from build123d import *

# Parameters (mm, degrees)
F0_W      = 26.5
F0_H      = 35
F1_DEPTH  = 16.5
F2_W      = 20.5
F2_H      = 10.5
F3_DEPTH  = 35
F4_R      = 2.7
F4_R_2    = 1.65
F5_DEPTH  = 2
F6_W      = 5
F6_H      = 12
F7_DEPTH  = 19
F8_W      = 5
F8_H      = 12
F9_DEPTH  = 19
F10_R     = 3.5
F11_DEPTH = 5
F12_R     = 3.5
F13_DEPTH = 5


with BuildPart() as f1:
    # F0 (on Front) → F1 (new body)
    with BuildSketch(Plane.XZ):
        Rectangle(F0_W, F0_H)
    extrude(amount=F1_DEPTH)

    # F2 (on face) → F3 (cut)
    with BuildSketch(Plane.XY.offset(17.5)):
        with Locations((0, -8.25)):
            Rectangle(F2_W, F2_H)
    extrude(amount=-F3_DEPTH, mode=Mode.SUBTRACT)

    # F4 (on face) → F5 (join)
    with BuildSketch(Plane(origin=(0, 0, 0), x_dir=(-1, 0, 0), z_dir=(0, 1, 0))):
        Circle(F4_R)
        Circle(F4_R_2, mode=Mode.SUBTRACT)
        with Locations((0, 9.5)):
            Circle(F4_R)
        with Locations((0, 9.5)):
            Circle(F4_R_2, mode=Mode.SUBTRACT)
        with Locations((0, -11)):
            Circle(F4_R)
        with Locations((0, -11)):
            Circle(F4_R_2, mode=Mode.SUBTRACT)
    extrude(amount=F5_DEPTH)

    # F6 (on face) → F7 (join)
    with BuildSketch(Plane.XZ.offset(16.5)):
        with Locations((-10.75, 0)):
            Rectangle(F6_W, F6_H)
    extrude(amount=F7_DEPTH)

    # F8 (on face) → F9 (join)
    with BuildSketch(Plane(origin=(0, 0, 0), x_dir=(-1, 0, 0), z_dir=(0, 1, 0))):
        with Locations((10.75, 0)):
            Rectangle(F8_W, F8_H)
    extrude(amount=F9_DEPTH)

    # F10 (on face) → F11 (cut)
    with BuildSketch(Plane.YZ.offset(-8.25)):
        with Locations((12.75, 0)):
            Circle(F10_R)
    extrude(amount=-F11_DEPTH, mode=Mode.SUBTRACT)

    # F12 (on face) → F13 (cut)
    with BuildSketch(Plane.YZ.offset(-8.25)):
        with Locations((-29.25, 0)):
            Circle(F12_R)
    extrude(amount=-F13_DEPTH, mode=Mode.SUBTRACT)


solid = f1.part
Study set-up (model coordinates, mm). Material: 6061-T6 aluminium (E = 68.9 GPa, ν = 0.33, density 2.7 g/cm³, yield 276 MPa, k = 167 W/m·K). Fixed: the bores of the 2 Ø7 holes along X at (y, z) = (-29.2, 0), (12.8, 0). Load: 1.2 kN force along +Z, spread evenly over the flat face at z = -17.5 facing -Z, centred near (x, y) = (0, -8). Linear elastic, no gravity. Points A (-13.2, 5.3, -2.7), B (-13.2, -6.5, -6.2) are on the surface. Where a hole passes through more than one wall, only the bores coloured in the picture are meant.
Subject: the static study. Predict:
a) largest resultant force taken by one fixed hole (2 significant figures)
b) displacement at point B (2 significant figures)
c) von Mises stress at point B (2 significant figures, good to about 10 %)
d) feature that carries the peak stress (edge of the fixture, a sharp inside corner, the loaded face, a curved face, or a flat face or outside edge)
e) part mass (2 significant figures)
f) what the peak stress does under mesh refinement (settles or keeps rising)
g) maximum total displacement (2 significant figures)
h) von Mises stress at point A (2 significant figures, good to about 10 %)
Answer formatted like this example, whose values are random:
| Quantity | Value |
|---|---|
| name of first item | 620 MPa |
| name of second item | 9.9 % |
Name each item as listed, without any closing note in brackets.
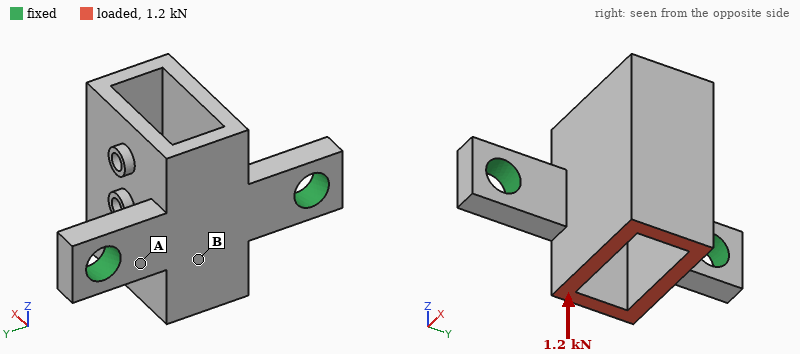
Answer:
| Quantity | Value |
|---|---|
| largest resultant force taken by one fixed hole | 600 N |
| displacement at point B | 0.041 mm |
| von Mises stress at point B | 21 MPa |
| feature that carries the peak stress | edge of the fixture |
| part mass | 26 g |
| what the peak stress does under mesh refinement | keeps rising |
| maximum total displacement | 0.21 mm |
| von Mises stress at point A | 86 MPa |
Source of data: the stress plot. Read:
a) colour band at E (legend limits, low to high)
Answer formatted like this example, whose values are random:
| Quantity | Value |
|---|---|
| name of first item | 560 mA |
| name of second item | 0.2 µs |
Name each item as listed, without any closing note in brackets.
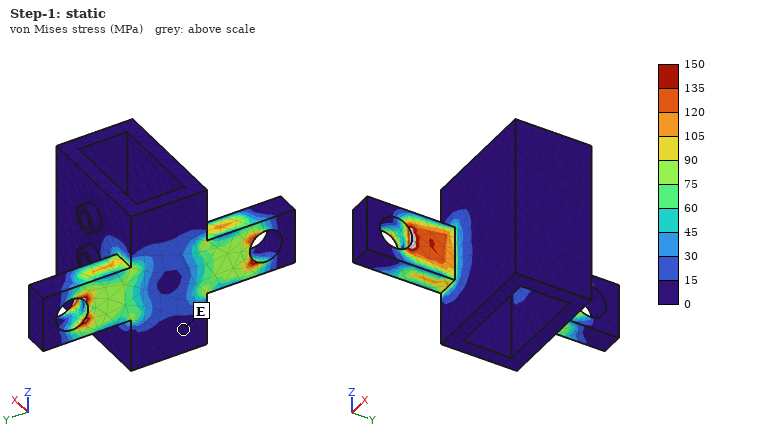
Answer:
| Quantity | Value |
|---|---|
| colour band at E | 0 to 15 MPa |
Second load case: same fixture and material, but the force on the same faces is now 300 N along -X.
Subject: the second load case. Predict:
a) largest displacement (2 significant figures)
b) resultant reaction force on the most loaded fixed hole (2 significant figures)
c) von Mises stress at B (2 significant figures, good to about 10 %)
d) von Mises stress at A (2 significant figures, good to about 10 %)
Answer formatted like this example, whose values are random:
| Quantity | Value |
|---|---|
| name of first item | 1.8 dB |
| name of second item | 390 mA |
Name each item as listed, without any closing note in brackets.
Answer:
| Quantity | Value |
|---|---|
| largest displacement | 86 µm |
| resultant reaction force on the most loaded fixed hole | 160 N |
| von Mises stress at B | 11 MPa |
| von Mises stress at A | 46 MPa |
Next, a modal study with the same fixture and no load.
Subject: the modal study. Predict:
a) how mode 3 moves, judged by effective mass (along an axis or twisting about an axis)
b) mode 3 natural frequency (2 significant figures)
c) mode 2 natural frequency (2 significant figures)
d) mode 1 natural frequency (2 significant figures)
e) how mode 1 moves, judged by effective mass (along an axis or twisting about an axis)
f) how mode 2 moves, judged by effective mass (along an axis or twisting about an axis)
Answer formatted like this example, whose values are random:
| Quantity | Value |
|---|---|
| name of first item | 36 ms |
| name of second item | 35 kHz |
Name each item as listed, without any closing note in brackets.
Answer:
| Quantity | Value |
|---|---|
| how mode 3 moves, judged by effective mass | along X |
| mode 3 natural frequency | 7600 Hz |
| mode 2 natural frequency | 4800 Hz |
| mode 1 natural frequency | 2800 Hz |
| how mode 1 moves, judged by effective mass | along Z |
| how mode 2 moves, judged by effective mass | along Y |
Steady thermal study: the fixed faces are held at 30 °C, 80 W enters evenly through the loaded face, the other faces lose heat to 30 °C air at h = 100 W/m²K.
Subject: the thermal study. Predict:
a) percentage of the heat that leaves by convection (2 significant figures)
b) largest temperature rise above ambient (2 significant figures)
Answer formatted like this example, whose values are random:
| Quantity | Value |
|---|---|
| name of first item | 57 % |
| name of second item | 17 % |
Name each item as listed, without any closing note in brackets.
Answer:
| Quantity | Value |
|---|---|
| percentage of the heat that leaves by convection | 32 % |
| largest temperature rise above ambient | 78 K |
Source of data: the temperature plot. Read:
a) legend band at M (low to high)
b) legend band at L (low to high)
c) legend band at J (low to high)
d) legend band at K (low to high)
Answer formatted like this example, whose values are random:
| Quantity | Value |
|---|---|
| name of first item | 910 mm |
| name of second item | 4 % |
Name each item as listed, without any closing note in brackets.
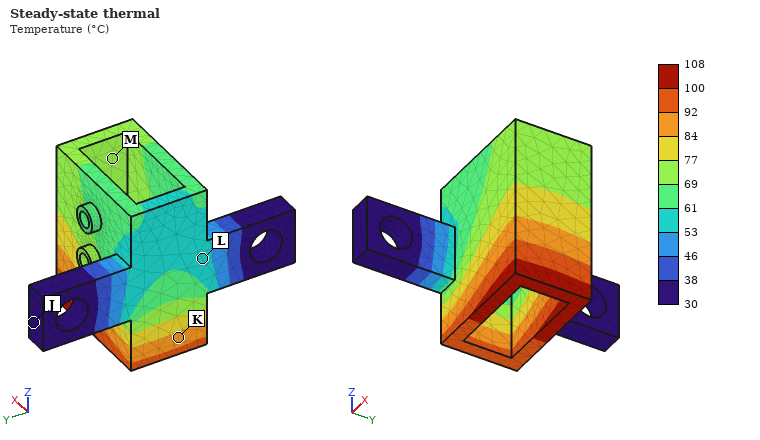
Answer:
| Quantity | Value |
|---|---|
| legend band at M | 69 to 77 °C |
| legend band at L | 53 to 61 °C |
| legend band at J | 30 to 38 °C |
| legend band at K | 84 to 92 °C |
